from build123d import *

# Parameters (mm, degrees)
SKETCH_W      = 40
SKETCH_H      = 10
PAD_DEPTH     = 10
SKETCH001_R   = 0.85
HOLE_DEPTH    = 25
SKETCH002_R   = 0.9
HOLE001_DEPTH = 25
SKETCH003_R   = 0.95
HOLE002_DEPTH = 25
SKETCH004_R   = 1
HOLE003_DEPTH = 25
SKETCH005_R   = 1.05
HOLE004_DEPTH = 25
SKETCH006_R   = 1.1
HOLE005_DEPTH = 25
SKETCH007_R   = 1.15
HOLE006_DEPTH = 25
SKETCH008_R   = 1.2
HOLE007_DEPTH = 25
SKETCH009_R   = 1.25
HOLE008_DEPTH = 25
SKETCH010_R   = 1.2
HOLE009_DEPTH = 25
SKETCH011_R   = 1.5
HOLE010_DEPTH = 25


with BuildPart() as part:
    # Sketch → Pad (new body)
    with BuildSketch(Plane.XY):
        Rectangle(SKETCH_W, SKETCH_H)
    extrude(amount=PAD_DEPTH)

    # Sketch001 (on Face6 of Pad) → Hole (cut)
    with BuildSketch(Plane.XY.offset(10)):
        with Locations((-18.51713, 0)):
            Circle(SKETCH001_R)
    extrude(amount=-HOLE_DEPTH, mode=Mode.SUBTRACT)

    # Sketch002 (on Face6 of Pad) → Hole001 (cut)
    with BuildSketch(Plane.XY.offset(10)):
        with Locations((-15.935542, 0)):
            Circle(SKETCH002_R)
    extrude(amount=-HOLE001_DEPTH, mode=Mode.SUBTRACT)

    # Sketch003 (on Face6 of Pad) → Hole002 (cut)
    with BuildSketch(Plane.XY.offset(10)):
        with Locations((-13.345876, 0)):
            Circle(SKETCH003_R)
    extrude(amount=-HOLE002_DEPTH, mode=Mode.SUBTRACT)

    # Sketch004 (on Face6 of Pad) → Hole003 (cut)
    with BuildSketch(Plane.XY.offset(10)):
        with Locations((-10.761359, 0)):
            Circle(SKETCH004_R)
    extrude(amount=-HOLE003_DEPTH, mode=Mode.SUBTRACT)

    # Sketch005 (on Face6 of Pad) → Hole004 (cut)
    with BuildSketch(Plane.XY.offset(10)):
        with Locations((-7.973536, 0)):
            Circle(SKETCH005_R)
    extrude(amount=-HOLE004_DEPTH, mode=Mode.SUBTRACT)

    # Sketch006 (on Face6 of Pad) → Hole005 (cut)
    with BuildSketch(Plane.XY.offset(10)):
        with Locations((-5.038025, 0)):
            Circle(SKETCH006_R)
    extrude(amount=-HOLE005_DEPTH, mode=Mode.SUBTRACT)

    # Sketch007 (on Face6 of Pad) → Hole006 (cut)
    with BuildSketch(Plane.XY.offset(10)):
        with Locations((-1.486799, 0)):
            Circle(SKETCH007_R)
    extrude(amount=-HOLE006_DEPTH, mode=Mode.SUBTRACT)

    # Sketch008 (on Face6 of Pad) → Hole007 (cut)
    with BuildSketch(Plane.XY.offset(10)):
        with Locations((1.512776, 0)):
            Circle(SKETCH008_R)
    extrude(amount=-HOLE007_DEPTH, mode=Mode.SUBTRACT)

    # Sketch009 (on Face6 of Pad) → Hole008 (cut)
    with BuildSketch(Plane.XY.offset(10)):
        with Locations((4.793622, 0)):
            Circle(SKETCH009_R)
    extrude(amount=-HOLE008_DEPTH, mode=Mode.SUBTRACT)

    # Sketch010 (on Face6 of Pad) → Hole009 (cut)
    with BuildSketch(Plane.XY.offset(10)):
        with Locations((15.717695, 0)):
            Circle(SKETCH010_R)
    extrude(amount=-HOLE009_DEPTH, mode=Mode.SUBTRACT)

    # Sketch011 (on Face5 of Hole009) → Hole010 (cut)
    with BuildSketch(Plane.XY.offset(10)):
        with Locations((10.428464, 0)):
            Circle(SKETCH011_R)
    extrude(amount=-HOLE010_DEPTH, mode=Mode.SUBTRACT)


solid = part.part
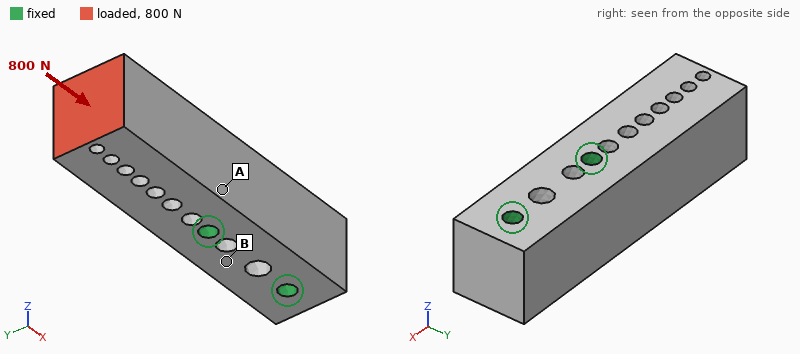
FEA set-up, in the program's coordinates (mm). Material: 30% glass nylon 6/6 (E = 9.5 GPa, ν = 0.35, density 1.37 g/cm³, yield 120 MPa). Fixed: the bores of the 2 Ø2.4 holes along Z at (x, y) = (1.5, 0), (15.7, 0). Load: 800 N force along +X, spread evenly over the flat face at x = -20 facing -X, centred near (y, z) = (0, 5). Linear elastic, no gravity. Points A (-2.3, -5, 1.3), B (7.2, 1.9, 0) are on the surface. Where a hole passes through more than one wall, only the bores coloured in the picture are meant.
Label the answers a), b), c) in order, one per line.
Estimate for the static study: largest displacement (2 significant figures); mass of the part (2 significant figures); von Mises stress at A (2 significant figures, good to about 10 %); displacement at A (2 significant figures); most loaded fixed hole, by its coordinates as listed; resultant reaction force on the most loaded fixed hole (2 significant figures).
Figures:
a) 28 µm
b) 4.9 g
c) 6.4 MPa
d) 7.2 µm
e) (1.5, 0)
f) 670 N
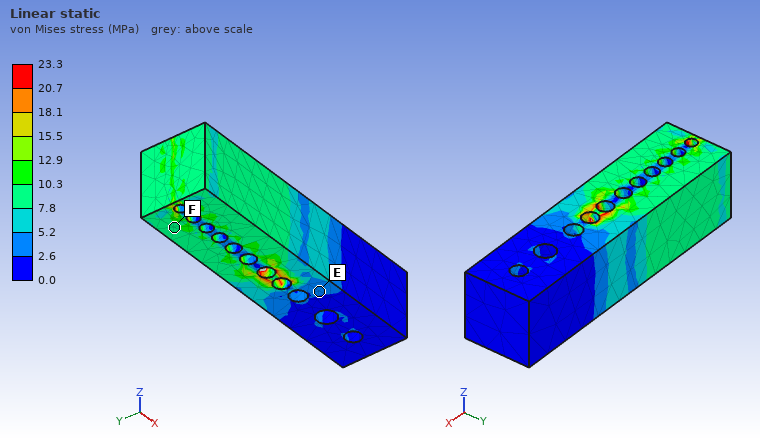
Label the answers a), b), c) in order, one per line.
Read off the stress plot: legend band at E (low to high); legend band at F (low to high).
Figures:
a) 2.6 to 5.2 MPa
b) 7.8 to 10.3 MPa
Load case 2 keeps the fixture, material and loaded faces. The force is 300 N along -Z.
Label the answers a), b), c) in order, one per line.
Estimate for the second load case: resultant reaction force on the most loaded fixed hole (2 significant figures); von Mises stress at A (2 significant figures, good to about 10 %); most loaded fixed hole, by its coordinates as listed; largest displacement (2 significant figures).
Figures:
a) 420 N
b) 22 MPa
c) (1.5, 0)
d) 0.22 mm
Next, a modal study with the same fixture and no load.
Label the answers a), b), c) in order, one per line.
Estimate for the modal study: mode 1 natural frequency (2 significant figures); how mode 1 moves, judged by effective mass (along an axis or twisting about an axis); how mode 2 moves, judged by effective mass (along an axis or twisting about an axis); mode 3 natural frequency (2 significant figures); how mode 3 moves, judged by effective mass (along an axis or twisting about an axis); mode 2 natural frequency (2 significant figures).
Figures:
a) 6100 Hz
b) along Y
c) along Z
d) 15 kHz
e) twisting about X
f) 7000 Hz
